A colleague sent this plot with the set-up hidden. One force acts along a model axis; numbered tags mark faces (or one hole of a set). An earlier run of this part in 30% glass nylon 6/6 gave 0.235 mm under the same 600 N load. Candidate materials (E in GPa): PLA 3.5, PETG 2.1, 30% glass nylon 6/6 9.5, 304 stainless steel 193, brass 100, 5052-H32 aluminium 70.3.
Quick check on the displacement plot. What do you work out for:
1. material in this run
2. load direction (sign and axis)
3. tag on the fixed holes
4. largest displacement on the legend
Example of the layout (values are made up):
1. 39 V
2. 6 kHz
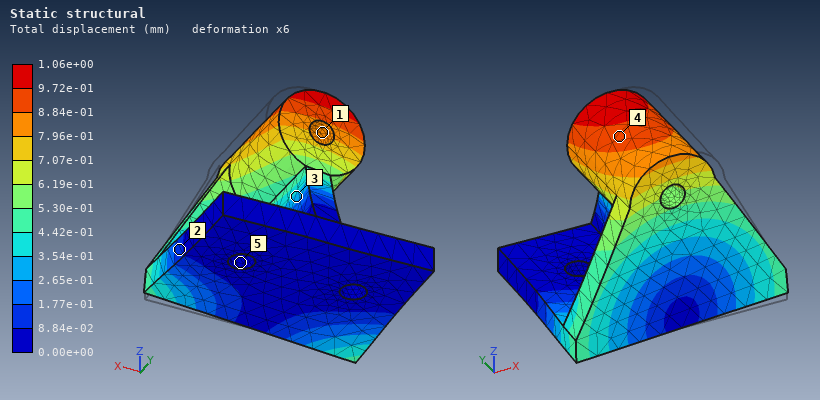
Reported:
1. PETG
2. -X
3. 5
4. 1.06e+00 mm
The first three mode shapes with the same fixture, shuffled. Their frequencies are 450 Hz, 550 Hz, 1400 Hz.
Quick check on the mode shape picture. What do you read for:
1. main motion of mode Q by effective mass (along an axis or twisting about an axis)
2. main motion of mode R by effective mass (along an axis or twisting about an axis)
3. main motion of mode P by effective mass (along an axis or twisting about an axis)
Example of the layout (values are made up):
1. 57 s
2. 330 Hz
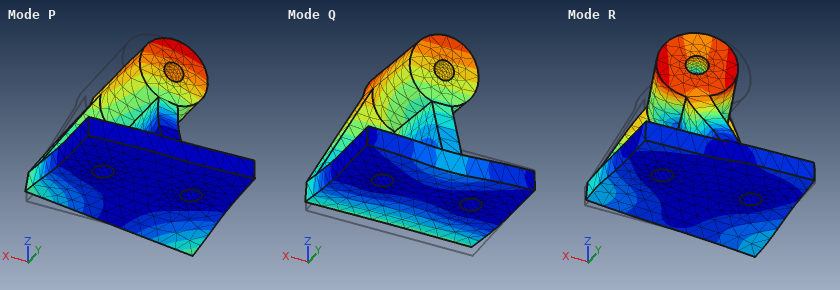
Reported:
1. along Y
2. twisting about Z
3. along X
